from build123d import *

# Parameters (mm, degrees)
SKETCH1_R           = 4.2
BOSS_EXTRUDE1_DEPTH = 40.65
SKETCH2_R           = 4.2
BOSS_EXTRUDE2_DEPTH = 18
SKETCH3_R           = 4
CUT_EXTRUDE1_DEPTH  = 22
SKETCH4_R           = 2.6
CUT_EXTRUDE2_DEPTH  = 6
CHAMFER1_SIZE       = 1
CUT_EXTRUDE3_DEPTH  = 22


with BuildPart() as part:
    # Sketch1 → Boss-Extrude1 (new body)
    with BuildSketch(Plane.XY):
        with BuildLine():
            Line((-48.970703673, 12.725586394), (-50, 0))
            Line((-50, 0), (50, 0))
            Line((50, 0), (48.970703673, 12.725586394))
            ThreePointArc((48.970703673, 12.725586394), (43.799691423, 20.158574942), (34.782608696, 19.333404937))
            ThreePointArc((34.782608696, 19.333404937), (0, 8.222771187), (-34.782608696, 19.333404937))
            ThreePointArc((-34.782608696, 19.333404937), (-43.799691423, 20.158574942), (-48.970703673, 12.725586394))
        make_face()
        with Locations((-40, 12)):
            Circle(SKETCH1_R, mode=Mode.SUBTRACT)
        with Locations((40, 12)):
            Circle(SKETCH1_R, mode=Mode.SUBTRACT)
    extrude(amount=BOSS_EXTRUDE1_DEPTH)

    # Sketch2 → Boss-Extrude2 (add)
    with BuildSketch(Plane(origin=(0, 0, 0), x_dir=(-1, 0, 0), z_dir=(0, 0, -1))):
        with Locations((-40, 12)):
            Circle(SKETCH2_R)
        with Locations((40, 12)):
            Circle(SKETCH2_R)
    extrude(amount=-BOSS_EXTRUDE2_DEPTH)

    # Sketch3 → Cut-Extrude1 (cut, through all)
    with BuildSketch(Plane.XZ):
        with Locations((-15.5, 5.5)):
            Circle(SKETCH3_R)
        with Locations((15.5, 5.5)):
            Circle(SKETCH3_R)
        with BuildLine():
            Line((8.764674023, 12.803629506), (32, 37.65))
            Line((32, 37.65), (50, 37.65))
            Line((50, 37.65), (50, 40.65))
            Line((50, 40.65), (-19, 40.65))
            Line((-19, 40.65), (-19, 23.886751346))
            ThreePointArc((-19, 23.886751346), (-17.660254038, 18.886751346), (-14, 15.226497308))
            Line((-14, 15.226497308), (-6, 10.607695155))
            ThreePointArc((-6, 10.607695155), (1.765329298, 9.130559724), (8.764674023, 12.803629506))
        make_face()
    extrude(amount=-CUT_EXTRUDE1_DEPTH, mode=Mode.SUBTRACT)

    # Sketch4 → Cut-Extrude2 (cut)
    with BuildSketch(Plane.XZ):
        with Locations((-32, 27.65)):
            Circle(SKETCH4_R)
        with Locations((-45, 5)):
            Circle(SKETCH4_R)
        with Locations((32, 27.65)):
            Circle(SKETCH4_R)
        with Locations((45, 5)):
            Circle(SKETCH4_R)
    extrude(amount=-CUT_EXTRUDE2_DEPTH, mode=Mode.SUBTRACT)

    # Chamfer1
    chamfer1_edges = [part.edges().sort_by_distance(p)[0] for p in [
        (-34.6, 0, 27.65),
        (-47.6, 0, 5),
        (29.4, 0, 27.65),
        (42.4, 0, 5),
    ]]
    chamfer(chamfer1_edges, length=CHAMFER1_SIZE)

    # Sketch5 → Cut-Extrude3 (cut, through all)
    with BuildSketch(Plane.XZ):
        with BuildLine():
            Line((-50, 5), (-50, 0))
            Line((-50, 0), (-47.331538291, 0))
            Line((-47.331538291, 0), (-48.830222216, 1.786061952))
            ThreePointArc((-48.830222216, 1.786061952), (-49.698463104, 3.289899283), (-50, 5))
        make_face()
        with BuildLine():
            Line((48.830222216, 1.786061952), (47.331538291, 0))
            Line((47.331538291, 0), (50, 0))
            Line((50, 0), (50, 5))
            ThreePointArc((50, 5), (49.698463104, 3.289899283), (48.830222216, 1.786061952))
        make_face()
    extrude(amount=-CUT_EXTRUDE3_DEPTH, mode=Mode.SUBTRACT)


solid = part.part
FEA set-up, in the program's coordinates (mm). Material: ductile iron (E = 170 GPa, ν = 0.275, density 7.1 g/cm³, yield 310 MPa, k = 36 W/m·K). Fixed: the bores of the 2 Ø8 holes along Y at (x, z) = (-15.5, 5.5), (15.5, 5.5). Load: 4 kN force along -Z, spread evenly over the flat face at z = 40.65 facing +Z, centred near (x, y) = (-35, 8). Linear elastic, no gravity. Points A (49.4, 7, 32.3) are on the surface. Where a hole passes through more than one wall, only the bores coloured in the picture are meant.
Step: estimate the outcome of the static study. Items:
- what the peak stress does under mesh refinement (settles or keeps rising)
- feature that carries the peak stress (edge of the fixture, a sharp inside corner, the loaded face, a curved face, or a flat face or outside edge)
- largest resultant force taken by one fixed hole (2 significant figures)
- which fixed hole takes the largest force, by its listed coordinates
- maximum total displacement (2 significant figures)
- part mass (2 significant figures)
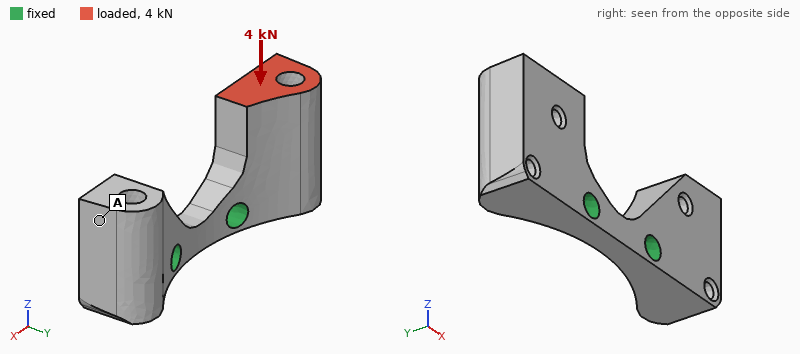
keeps rising
edge of the fixture
4.3 kN
(-15.5, 5.5)
52 µm
290 g
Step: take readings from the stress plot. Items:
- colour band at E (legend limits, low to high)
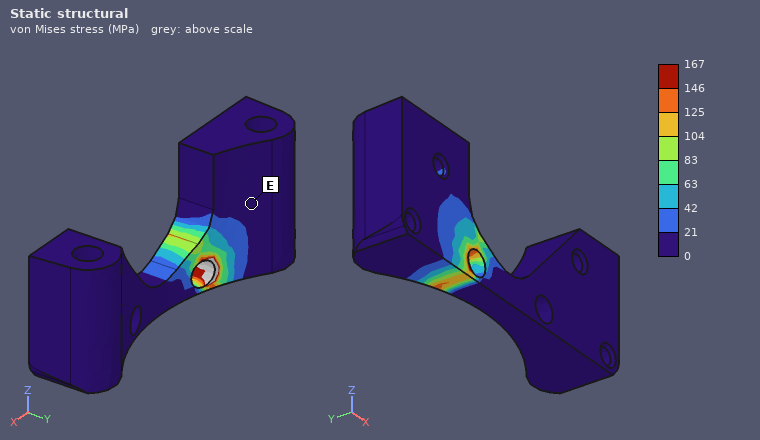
0 to 21 MPa
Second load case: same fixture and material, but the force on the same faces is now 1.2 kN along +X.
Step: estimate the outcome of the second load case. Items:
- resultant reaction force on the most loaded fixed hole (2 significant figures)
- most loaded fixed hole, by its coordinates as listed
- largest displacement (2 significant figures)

1.1 kN
(-15.5, 5.5)
34 µm
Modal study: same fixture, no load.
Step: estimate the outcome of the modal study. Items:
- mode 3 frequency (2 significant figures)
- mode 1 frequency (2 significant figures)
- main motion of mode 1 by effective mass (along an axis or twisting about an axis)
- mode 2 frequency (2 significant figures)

4200 Hz
3700 Hz
along Y
4100 Hz
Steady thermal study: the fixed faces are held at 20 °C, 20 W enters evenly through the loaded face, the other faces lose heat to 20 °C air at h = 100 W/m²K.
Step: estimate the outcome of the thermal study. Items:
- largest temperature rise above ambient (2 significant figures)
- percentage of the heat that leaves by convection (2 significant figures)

40 K
52 %
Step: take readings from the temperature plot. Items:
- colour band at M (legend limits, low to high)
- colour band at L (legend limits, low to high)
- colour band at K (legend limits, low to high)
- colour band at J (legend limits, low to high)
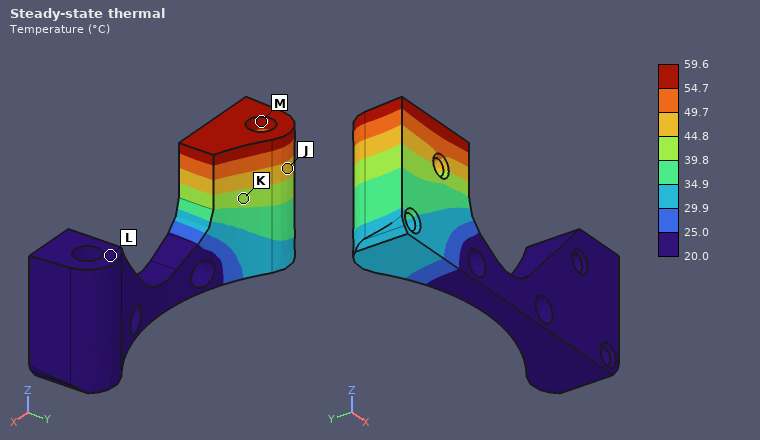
54.7 to 59.6 °C
20.0 to 25.0 °C
39.8 to 44.8 °C
44.8 to 49.7 °C
